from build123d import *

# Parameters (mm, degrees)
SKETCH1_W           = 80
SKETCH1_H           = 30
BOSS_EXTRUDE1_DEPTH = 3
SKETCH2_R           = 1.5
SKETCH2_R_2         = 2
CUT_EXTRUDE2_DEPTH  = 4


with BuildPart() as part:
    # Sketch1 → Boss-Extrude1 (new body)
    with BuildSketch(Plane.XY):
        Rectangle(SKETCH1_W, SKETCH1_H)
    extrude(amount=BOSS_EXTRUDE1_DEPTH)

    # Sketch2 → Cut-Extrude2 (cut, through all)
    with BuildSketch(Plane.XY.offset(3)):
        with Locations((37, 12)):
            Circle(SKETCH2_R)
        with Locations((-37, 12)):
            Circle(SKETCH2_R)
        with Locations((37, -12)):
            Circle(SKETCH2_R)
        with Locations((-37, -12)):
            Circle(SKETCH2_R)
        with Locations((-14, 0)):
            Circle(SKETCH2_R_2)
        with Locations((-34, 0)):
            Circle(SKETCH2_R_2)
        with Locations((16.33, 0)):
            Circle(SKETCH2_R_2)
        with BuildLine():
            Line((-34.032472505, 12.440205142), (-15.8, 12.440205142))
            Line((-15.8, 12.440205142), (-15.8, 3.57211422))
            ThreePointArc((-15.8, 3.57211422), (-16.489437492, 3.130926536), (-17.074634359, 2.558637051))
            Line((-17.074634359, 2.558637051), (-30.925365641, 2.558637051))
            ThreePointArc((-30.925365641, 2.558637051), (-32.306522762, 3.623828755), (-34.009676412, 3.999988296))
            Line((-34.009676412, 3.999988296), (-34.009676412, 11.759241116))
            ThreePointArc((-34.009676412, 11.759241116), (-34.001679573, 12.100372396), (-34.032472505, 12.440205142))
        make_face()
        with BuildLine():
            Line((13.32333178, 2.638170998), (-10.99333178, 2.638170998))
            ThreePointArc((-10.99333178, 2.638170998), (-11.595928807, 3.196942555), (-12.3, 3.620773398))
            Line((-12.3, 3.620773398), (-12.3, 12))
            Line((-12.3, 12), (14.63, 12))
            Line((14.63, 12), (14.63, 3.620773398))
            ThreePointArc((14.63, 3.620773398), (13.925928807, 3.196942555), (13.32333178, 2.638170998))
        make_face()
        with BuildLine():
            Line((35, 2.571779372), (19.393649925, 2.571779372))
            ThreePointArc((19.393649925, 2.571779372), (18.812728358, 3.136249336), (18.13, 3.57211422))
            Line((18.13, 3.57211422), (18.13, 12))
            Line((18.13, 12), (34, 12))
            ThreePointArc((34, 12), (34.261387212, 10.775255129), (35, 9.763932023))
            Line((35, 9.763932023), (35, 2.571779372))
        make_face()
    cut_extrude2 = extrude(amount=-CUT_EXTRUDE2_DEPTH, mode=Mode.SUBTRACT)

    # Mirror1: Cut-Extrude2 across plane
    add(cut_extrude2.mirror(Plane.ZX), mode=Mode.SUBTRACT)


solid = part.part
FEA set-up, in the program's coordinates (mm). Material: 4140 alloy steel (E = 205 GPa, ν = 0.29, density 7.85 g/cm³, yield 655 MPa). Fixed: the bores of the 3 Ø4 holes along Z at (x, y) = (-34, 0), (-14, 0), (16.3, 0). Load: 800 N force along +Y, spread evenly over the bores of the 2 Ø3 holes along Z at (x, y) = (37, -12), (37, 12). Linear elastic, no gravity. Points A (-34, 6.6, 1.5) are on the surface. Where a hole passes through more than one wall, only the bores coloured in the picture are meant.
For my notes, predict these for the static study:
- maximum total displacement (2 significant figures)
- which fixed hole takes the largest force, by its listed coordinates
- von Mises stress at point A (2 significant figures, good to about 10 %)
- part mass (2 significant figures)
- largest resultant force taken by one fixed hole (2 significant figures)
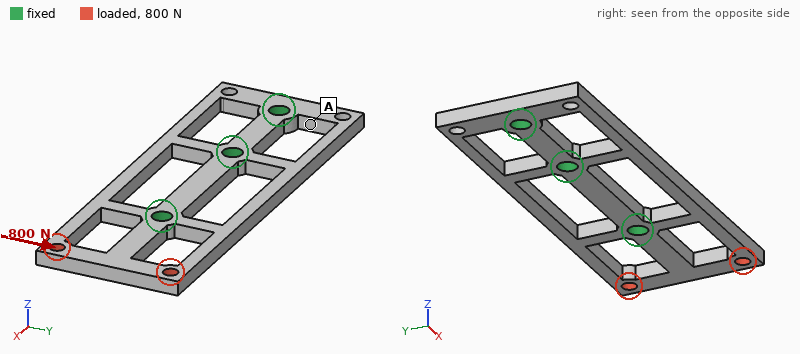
87 µm
(16.3, 0)
35 MPa
27 g
880 N
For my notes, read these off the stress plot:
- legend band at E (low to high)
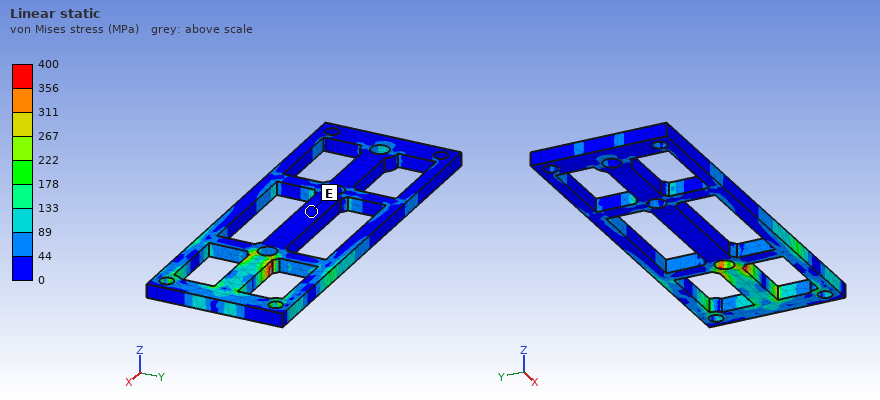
0 to 44 MPa
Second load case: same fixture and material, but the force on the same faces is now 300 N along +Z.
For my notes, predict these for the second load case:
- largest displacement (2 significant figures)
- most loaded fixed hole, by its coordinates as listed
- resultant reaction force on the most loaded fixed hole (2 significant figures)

0.25 mm
(16.3, 0)
340 N
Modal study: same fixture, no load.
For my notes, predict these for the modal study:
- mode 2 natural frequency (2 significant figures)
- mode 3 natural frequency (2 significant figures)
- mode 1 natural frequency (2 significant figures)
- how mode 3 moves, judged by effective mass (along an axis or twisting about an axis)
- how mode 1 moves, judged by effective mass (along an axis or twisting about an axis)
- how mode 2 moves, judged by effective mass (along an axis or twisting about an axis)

4500 Hz
6400 Hz
3000 Hz
along Z
along Z
twisting about X
